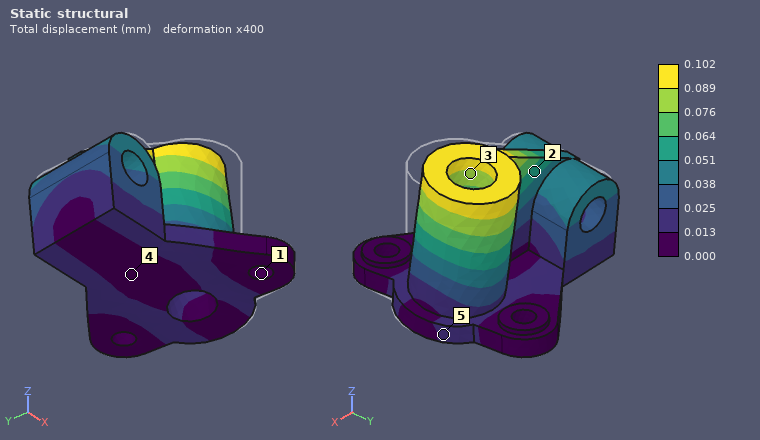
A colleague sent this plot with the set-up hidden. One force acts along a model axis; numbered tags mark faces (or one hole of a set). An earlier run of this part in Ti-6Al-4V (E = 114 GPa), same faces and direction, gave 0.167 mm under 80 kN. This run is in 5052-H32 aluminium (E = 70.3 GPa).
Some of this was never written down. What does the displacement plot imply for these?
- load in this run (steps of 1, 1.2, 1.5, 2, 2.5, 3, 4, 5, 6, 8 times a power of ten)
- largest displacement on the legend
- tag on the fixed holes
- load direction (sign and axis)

30 kN
0.102 mm
1
+Y
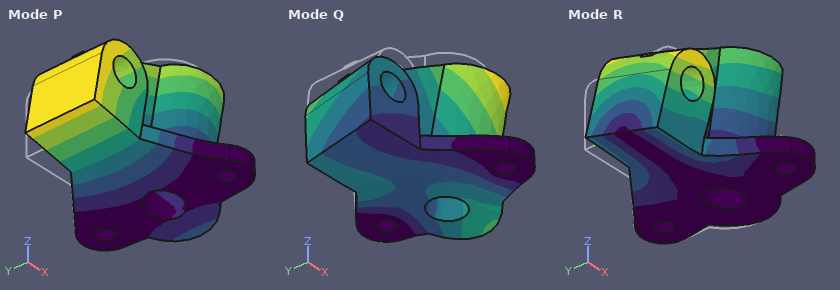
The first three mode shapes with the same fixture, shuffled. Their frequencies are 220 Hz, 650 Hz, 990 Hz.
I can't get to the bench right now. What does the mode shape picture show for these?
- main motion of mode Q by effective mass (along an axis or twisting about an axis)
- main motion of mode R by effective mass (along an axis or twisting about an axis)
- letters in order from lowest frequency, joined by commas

along Z
along Y
P, R, Q
